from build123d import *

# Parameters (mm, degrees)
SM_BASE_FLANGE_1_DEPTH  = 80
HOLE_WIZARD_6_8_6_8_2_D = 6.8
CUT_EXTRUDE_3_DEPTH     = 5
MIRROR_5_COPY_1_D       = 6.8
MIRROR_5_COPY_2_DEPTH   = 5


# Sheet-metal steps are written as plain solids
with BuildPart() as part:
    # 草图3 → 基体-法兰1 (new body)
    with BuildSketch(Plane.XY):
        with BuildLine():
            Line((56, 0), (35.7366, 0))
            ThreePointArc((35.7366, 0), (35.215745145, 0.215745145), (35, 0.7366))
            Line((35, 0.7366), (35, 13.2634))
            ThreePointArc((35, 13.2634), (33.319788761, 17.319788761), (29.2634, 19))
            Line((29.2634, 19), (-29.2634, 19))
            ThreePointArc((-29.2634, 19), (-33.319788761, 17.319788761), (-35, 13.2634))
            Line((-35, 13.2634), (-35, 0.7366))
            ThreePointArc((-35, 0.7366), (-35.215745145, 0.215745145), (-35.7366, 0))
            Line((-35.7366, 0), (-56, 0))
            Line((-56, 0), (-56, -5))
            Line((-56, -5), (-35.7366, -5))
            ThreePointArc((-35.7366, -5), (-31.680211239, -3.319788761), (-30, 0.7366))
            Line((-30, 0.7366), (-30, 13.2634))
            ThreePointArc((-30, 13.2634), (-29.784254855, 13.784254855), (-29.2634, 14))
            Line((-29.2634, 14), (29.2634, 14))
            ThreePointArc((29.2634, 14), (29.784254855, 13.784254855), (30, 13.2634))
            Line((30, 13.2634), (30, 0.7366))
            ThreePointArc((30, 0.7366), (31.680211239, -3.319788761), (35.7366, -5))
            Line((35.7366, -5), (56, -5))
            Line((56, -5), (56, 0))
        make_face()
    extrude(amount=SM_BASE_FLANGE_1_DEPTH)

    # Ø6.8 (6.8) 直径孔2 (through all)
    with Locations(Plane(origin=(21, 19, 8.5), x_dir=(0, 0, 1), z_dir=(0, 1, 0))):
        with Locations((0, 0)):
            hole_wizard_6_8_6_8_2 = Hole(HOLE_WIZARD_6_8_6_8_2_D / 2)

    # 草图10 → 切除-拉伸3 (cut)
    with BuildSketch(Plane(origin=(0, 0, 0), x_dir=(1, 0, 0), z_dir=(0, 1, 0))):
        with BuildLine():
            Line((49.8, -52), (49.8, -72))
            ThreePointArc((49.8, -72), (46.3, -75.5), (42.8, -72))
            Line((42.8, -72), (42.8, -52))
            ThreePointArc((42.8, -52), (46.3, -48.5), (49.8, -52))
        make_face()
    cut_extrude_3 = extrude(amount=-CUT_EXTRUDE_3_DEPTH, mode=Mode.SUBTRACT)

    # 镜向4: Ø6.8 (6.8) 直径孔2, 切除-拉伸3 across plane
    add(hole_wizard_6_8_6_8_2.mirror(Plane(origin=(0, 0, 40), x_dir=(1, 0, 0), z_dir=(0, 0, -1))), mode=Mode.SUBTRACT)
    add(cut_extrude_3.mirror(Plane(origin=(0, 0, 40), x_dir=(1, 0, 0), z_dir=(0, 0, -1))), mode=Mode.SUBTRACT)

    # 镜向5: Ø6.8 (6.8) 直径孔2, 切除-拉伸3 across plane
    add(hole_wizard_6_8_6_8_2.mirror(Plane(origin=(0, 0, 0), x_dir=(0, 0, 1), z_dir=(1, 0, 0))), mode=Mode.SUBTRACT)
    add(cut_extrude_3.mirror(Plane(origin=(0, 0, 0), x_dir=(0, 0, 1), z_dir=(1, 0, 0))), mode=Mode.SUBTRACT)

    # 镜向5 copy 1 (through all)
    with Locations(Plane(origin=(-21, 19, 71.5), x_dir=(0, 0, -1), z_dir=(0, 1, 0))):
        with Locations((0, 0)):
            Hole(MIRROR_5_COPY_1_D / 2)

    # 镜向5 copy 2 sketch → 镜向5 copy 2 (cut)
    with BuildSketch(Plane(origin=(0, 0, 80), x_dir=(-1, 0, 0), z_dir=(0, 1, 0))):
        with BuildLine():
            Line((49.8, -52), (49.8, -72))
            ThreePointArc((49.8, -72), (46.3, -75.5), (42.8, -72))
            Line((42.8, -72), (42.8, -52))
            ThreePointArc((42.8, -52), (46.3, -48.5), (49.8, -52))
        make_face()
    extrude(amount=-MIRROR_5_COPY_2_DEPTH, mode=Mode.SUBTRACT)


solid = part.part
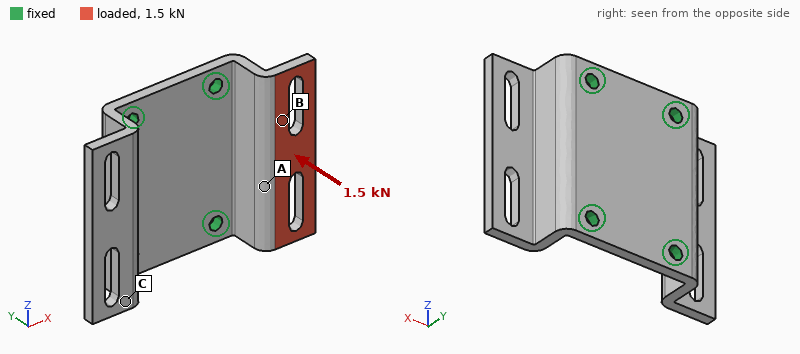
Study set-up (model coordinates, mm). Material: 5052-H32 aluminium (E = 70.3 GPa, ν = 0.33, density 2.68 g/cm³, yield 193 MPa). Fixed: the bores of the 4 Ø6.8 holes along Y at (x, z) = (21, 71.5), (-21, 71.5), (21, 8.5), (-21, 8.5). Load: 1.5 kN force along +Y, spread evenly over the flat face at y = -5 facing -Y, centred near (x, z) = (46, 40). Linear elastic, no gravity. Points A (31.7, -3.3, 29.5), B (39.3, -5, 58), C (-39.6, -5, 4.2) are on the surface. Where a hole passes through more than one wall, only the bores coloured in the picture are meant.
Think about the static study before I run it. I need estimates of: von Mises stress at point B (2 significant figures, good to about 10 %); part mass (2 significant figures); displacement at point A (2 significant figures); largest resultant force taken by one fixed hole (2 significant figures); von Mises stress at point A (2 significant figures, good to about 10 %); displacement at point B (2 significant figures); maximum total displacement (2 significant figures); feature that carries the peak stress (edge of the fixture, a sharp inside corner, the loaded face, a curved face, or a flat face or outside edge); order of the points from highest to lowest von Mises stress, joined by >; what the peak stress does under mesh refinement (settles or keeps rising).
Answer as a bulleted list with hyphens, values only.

- 19 MPa
- 140 g
- 0.17 mm
- 940 N
- 36 MPa
- 0.22 mm
- 0.43 mm
- edge of the fixture
- A > B > C
- keeps rising
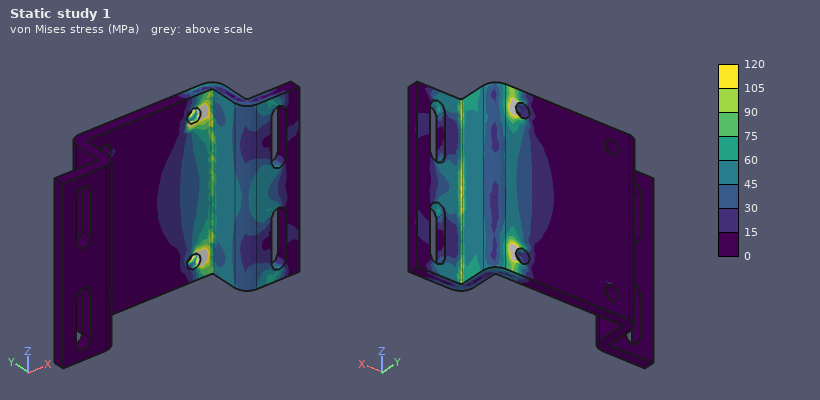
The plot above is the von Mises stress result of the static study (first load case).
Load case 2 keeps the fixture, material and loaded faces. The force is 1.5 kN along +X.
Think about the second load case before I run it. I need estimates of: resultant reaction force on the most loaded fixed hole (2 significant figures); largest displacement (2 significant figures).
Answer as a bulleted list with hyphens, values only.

- 560 N
- 0.38 mm
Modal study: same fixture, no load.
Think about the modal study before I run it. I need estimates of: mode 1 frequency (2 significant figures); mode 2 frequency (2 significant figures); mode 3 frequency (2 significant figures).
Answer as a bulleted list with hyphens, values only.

- 2200 Hz
- 2200 Hz
- 3700 Hz
